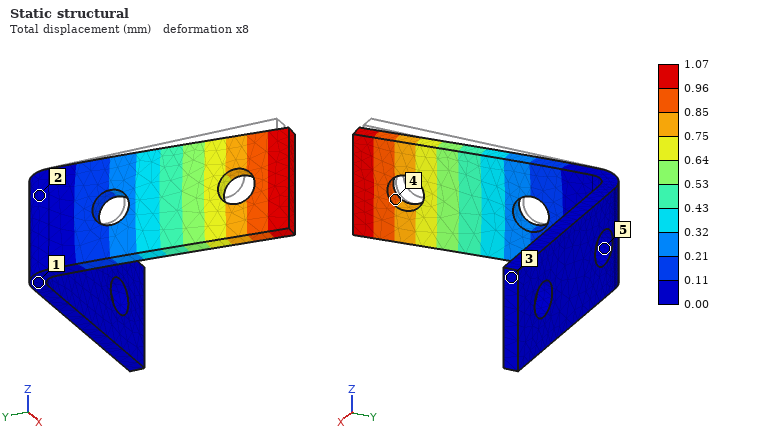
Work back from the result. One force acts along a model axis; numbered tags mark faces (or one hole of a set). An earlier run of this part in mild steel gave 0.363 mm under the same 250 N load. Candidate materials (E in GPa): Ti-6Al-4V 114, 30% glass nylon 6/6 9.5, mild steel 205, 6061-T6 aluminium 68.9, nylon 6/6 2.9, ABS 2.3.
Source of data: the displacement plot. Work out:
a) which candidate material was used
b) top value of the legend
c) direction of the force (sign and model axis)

6061-T6 aluminium
1.07 mm
+X
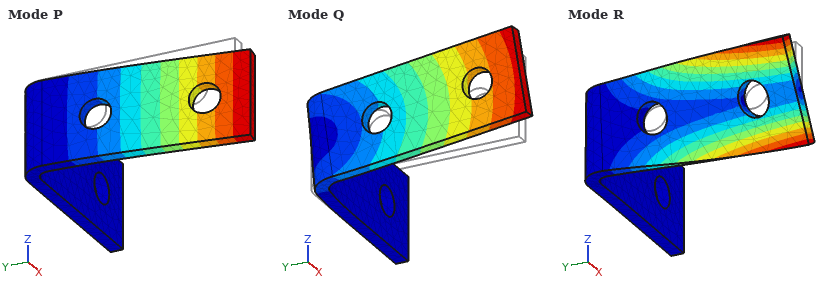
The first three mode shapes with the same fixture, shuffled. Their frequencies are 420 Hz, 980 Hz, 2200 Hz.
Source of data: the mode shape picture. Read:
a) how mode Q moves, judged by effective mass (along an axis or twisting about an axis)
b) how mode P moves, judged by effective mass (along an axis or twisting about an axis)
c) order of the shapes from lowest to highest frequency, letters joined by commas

along Z
along X
P, Q, R
